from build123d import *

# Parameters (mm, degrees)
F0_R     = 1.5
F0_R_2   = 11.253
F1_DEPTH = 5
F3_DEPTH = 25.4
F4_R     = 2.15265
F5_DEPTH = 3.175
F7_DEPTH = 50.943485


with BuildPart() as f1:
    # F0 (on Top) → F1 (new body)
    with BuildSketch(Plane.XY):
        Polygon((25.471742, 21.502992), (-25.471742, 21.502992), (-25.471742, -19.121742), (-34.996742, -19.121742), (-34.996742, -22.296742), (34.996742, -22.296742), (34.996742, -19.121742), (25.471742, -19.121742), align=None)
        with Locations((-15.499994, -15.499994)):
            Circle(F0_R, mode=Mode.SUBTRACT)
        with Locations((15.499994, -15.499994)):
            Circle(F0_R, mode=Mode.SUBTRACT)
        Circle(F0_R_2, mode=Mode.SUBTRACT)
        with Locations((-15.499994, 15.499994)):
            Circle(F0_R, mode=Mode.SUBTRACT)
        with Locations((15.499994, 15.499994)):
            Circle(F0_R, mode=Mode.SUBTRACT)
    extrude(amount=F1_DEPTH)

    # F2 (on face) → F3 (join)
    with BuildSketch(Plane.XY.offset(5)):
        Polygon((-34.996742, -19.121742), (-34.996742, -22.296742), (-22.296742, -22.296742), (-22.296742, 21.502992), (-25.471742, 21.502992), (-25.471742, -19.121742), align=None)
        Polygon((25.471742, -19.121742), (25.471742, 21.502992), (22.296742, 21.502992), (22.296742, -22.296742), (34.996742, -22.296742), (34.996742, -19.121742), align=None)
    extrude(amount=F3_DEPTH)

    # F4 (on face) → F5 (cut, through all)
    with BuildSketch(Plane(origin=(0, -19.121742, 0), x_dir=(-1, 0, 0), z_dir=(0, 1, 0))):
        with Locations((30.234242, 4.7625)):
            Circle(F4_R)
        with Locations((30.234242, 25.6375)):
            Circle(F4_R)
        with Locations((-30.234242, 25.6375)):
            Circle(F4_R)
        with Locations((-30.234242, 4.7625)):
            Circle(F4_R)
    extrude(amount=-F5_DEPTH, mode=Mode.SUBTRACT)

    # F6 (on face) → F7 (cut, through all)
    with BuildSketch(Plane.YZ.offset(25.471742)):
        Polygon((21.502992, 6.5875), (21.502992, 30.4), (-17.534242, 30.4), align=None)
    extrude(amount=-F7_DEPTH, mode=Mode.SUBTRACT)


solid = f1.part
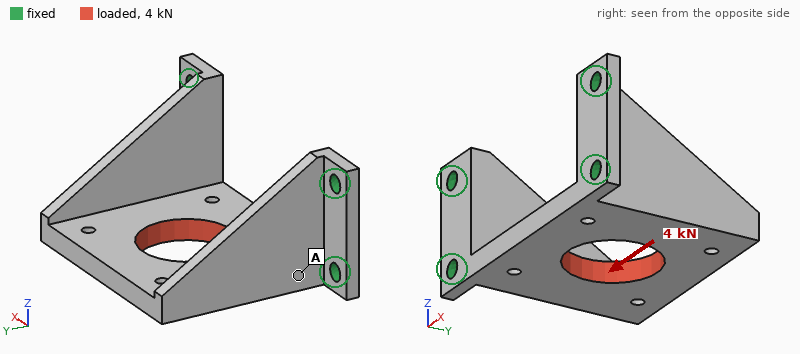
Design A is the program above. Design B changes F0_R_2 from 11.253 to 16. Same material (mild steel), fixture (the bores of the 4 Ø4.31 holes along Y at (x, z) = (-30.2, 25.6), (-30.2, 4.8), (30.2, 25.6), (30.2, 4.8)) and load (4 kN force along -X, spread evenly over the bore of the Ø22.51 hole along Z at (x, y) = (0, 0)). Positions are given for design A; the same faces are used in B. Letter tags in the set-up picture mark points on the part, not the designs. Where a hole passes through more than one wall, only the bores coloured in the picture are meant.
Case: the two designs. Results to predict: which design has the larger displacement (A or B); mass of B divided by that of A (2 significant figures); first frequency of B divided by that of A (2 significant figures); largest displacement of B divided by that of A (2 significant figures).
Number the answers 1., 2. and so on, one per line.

1. B
2. 0.86
3. 1.1
4. 1.9
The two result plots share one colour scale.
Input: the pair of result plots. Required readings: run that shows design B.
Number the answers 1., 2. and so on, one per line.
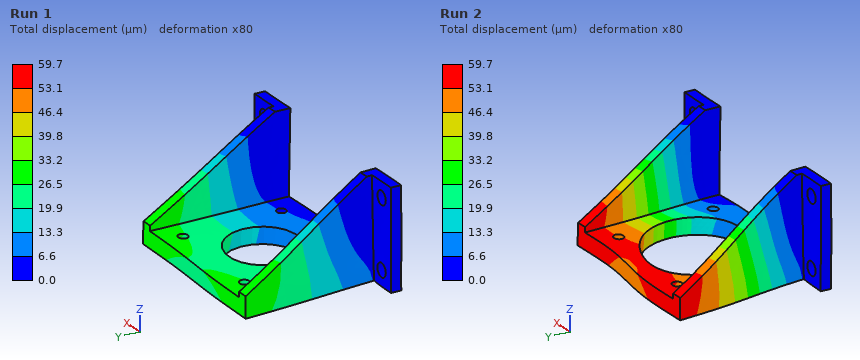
1. Run 2
